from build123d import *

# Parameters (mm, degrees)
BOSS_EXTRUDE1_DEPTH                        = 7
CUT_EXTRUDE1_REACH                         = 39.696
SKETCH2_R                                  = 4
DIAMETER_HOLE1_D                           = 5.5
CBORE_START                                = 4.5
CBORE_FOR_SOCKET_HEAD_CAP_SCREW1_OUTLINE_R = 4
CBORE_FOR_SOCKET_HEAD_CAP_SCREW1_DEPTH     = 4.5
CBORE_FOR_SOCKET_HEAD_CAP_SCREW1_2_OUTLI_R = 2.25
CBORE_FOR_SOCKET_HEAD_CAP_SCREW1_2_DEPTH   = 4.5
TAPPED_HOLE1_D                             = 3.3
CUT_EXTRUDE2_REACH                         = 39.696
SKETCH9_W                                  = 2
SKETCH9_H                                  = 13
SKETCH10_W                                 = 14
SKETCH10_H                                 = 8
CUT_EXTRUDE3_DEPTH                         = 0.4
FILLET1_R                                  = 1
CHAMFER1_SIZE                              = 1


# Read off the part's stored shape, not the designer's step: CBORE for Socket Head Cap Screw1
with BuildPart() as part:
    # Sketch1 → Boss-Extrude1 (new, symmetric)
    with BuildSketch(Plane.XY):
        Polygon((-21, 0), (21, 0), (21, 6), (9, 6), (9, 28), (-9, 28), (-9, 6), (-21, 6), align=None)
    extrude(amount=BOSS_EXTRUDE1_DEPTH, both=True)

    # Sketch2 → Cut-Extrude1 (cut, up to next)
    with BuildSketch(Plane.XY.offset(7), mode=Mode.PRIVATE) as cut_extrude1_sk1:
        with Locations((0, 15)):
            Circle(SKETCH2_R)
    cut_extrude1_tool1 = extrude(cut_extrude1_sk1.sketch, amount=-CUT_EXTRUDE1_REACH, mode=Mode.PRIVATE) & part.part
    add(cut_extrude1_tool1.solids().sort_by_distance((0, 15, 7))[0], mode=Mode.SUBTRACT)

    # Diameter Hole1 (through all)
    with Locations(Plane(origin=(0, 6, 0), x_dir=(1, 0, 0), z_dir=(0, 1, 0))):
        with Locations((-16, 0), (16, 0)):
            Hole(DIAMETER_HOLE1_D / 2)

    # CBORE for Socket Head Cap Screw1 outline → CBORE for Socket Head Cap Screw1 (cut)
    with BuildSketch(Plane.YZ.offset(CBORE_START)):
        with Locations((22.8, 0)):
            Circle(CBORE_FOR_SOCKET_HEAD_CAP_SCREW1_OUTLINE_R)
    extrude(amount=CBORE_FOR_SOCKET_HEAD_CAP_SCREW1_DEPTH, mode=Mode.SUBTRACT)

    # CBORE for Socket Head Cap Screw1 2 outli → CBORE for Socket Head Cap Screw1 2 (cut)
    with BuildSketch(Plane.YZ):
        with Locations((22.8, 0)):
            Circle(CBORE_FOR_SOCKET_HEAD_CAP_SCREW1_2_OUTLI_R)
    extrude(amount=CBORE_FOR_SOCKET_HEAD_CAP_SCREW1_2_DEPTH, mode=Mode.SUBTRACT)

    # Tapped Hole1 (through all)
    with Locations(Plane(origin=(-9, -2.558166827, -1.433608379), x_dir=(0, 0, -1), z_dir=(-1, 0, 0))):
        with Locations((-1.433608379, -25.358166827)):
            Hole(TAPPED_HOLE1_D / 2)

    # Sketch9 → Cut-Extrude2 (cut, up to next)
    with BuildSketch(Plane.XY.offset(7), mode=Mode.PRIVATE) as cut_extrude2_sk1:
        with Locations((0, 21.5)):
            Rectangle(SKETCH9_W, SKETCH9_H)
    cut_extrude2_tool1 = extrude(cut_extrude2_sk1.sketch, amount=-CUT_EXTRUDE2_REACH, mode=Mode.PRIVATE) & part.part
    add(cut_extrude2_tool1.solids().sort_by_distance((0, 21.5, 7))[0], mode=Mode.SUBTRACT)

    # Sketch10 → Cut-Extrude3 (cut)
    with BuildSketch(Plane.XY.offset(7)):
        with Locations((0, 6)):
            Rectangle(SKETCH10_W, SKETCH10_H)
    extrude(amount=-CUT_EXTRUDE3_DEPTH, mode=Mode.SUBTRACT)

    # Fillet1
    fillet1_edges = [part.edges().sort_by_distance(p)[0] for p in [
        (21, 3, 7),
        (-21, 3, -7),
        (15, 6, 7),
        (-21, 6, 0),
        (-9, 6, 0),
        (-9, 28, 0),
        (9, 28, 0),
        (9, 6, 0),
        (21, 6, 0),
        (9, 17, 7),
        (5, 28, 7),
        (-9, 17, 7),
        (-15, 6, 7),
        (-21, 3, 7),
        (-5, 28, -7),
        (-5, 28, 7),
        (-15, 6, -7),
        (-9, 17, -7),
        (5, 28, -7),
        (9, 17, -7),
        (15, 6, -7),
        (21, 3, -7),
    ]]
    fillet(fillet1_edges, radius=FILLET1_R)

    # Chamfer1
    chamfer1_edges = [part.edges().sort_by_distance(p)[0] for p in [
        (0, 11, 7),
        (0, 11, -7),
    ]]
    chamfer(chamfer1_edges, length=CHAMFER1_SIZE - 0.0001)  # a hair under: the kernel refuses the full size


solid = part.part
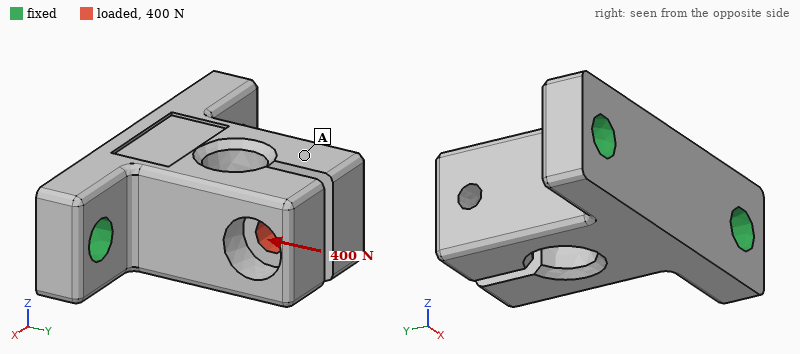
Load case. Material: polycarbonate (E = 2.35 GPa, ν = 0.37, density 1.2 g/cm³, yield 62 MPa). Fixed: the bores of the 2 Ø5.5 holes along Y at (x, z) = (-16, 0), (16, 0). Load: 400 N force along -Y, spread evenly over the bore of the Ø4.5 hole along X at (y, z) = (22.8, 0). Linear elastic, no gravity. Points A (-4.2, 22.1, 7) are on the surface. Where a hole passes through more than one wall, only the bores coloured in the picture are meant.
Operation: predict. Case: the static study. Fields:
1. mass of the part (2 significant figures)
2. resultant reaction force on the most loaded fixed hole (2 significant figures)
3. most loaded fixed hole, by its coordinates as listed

8.8 g
270 N
(16, 0)
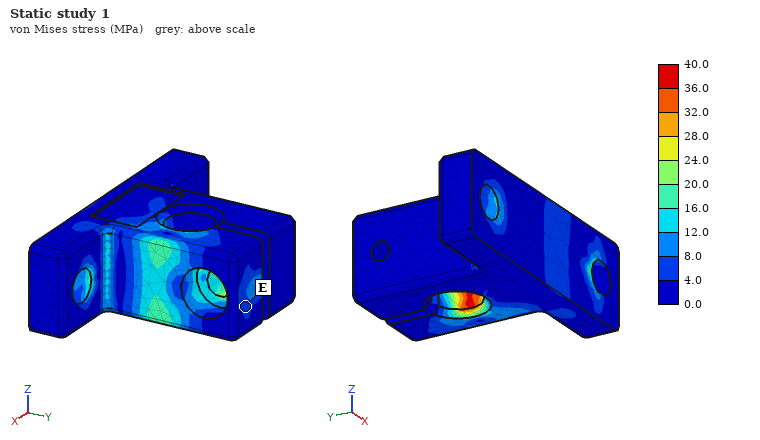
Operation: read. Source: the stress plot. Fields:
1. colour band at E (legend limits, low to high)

4.0 to 8.0 MPa
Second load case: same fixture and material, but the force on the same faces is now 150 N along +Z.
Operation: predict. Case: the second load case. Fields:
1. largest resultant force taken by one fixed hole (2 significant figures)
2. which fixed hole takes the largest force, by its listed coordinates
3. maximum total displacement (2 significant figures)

88 N
(16, 0)
0.61 mm
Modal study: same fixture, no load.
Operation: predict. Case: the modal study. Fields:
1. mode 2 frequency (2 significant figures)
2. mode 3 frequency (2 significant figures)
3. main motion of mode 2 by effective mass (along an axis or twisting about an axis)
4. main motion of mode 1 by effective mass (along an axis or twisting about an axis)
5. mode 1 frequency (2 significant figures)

2600 Hz
2800 Hz
along X
along Z
1900 Hz
